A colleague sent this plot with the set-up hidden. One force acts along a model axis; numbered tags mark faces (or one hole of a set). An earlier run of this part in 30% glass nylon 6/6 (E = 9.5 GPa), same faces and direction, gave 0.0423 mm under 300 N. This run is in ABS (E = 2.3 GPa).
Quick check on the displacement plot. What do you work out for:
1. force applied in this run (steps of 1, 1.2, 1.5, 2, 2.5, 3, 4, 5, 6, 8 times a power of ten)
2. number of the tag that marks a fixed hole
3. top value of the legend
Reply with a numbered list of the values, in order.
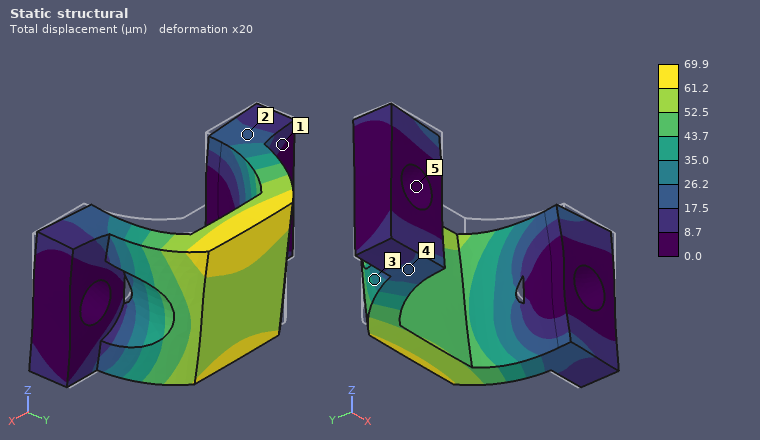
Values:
1. 120 N
2. 5
3. 69.9 µm
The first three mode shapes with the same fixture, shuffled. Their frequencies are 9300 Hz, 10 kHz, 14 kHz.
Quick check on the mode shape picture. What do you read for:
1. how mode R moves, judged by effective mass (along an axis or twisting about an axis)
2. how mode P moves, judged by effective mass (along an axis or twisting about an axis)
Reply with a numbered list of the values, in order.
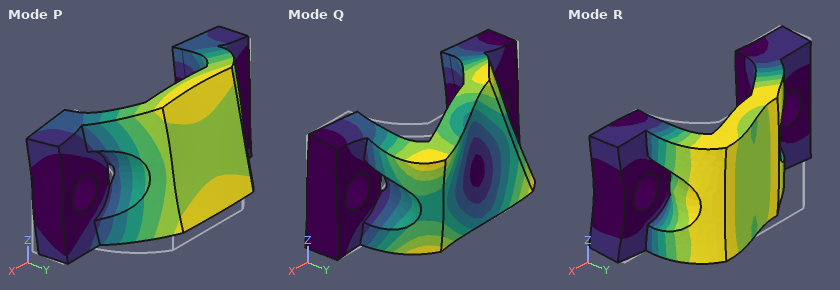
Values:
1. along X
2. along Z
